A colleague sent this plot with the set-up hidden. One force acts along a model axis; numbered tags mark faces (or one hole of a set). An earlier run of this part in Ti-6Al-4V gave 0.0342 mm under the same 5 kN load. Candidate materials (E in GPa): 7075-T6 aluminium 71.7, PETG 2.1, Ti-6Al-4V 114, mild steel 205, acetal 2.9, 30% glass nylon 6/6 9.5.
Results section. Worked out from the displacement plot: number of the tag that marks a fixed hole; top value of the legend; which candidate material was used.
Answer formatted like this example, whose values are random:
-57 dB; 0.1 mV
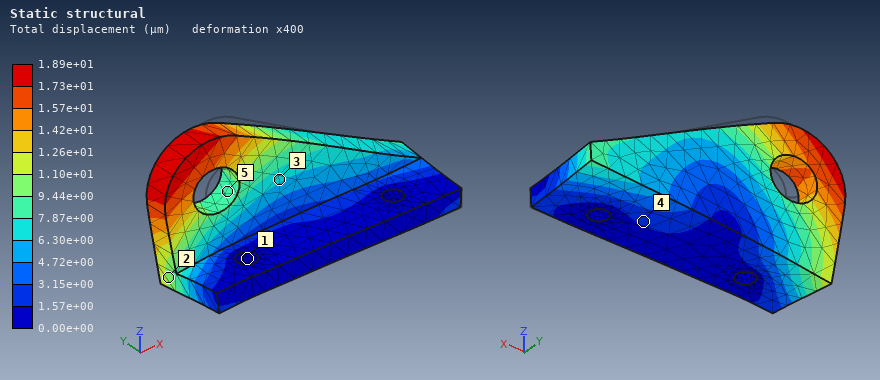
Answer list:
1; 1.89e+01 µm; mild steel
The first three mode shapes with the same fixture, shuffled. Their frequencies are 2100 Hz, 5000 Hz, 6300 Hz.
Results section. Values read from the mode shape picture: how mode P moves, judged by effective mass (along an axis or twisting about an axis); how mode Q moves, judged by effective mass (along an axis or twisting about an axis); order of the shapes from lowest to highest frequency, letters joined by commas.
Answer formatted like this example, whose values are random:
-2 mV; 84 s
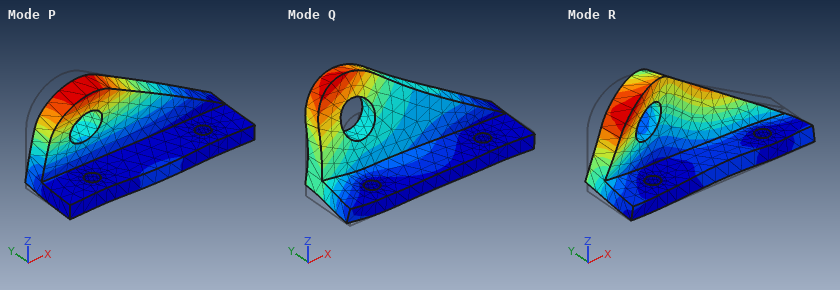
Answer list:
along Y; along Z; P, R, Q
